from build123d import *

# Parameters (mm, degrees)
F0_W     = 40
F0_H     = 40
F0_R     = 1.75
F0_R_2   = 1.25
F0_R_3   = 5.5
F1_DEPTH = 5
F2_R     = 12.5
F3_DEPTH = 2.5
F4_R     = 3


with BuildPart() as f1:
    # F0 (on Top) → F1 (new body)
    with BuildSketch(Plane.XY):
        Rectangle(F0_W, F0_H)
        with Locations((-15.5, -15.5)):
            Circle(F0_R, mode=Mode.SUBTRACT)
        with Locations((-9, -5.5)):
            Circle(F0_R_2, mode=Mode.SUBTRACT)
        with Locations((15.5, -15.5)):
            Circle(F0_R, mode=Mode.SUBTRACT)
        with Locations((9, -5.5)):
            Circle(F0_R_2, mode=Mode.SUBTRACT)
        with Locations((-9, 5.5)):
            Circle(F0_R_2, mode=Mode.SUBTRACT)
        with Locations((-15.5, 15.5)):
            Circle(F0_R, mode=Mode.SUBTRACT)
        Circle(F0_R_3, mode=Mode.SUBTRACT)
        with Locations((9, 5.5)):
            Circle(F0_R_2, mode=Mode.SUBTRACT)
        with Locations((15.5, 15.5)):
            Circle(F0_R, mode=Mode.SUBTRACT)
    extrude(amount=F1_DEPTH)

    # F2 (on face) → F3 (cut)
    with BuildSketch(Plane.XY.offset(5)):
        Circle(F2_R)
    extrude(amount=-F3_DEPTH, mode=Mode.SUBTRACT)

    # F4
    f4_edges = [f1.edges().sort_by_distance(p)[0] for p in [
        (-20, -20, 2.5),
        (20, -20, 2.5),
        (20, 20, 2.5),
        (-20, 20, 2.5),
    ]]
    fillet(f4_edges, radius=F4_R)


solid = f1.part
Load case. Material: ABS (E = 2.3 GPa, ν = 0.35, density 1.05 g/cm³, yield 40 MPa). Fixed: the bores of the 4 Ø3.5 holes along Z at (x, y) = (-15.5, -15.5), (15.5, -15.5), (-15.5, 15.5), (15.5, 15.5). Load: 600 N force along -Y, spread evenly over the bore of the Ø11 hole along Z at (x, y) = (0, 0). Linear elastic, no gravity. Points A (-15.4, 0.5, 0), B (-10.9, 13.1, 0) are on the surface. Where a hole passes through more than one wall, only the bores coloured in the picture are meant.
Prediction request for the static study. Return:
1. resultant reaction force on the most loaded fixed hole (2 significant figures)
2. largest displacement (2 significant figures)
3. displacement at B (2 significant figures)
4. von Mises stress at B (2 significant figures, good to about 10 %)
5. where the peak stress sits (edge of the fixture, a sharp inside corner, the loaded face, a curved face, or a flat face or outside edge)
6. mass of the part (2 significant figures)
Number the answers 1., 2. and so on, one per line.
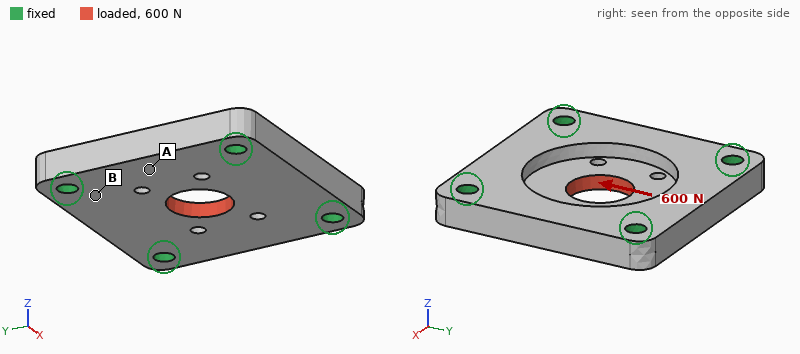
1. 160 N
2. 60 µm
3. 15 µm
4. 5.8 MPa
5. a curved face
6. 6.6 g
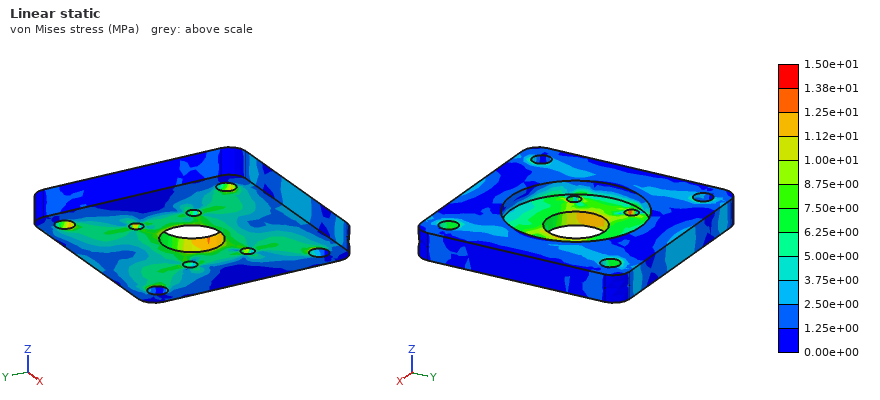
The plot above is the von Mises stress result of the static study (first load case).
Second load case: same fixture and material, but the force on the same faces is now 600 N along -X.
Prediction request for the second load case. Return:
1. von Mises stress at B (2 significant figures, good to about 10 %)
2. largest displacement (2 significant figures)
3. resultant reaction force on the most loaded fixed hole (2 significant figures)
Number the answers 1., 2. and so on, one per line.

1. 5.1 MPa
2. 60 µm
3. 160 N
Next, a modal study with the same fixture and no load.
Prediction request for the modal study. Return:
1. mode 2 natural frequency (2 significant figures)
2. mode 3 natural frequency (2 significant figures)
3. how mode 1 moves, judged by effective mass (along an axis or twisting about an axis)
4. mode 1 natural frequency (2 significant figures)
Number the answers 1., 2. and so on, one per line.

1. 7300 Hz
2. 7400 Hz
3. along Z
4. 5700 Hz
